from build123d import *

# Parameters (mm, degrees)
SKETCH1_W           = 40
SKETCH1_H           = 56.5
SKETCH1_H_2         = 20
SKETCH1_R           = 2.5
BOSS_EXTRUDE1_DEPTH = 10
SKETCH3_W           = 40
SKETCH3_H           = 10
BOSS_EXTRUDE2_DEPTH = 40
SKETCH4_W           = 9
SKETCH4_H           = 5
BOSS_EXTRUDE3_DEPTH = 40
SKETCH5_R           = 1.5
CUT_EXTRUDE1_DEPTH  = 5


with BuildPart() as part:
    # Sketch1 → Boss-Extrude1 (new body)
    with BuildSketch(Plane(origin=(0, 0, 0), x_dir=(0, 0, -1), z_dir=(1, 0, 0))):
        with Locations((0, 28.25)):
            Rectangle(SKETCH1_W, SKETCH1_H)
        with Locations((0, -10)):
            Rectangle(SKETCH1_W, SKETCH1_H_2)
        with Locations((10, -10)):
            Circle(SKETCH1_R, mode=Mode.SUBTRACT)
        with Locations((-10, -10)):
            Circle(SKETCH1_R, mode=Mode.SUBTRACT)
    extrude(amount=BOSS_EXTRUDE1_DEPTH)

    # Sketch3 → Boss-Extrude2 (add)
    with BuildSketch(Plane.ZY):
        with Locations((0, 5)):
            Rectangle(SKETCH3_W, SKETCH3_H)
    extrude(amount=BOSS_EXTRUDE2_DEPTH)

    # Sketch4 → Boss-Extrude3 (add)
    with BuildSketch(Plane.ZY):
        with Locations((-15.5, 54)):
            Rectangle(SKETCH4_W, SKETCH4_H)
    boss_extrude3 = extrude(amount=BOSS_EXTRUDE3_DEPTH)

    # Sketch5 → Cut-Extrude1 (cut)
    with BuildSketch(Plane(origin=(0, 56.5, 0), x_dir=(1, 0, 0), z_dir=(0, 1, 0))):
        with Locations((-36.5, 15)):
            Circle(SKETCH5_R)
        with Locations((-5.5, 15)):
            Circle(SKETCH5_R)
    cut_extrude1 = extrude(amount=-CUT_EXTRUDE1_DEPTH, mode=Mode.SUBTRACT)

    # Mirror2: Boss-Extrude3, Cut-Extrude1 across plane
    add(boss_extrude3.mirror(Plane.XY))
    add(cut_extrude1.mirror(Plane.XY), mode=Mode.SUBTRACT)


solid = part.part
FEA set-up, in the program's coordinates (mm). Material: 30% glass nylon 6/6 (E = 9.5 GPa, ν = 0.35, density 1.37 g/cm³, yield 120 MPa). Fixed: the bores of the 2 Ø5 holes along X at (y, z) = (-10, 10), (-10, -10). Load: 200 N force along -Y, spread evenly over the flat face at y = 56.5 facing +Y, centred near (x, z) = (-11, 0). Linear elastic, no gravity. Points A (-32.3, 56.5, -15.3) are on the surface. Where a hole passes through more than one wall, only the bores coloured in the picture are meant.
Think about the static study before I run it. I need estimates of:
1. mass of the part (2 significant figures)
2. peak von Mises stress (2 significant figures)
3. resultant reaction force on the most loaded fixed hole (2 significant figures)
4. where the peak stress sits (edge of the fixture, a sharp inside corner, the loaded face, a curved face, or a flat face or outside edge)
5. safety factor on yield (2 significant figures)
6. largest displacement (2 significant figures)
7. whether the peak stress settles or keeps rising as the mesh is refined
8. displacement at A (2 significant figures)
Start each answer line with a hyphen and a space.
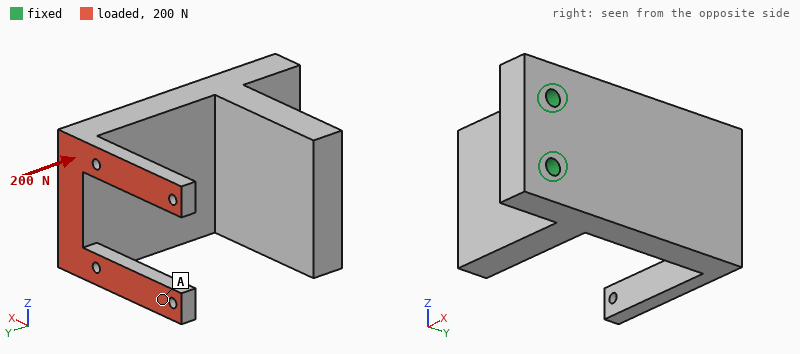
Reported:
- 68 g
- 64 MPa
- 100 N
- a curved face
- 1.9
- 1.1 mm
- settles
- 0.86 mm
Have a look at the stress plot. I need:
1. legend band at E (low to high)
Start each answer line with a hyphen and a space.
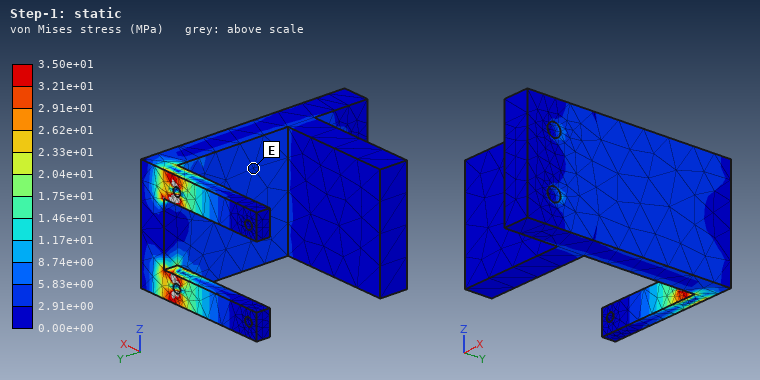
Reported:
- 2.91e+00 to 5.83e+00 MPa
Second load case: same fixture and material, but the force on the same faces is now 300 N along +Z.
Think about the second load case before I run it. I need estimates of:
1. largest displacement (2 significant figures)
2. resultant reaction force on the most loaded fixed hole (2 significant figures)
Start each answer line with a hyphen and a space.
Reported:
- 0.77 mm
- 890 N
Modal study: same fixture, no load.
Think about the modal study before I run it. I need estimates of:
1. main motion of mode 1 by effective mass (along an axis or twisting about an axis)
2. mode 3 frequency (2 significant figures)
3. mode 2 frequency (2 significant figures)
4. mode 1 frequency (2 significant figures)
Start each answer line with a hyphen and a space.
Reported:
- along X
- 1200 Hz
- 1100 Hz
- 710 Hz
